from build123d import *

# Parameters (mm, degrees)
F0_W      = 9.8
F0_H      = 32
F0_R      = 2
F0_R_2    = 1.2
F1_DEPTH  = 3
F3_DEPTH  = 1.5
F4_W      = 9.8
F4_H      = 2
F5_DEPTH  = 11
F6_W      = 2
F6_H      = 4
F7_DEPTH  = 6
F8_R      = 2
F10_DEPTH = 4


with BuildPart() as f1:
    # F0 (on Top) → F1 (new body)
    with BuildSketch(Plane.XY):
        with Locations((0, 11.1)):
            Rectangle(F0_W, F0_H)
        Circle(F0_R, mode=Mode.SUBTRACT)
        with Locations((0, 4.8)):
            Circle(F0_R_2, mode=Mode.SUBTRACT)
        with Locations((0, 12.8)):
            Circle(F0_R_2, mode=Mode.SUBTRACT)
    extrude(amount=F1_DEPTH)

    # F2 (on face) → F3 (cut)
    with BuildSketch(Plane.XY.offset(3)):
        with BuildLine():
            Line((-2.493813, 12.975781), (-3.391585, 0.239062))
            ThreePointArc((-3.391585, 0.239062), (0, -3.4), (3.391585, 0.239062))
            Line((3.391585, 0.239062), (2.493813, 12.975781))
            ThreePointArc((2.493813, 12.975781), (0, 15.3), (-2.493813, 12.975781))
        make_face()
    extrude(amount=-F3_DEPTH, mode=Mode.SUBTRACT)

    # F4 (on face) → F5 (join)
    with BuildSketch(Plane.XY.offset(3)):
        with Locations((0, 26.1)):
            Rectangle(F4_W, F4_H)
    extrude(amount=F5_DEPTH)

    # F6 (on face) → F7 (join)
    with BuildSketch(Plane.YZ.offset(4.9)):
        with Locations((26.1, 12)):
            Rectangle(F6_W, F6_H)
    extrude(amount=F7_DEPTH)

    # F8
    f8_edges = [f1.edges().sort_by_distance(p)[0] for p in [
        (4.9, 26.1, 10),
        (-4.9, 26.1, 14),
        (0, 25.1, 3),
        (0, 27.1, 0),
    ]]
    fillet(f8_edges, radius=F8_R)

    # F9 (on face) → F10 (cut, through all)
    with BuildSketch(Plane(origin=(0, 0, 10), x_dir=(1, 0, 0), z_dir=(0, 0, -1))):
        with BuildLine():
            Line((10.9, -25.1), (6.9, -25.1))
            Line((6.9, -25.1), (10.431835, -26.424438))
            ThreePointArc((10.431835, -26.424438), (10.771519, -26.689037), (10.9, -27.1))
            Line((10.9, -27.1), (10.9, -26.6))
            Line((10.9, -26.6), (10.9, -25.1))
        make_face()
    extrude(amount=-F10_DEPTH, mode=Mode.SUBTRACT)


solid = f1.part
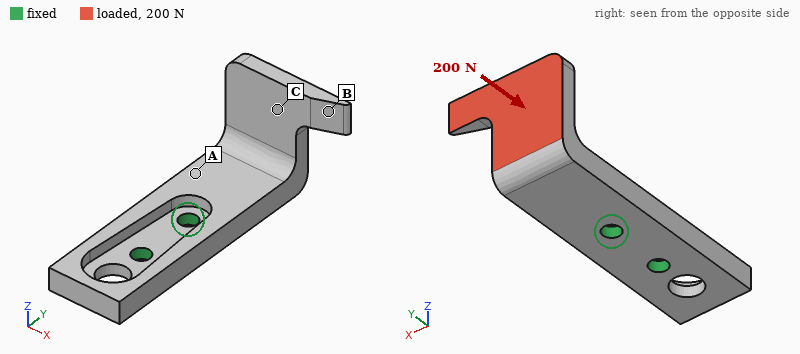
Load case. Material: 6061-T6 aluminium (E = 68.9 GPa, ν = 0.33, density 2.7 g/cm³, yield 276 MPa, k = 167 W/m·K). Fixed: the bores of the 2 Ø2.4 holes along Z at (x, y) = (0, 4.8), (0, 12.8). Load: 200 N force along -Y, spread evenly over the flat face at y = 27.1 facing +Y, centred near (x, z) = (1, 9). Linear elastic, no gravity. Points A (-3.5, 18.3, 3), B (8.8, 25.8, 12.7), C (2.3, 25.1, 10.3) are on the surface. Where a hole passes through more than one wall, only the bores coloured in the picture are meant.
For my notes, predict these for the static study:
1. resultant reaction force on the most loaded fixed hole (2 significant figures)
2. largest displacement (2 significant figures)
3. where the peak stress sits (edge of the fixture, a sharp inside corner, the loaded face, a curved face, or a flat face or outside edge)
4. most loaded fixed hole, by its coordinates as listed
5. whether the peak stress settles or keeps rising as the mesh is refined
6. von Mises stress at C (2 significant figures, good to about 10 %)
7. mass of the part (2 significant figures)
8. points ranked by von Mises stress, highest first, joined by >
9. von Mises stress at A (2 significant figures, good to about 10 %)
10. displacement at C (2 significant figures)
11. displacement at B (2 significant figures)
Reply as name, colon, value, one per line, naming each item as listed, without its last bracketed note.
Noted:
resultant reaction force on the most loaded fixed hole: 220 N
largest displacement: 0.35 mm
where the peak stress sits: edge of the fixture
most loaded fixed hole, by its coordinates as listed: (0, 4.8)
whether the peak stress settles or keeps rising as the mesh is refined: keeps rising
von Mises stress at C: 41 MPa
mass of the part: 2.7 g
points ranked by von Mises stress, highest first, joined by >: A > C > B
von Mises stress at A: 110 MPa
displacement at C: 0.21 mm
displacement at B: 0.30 mm
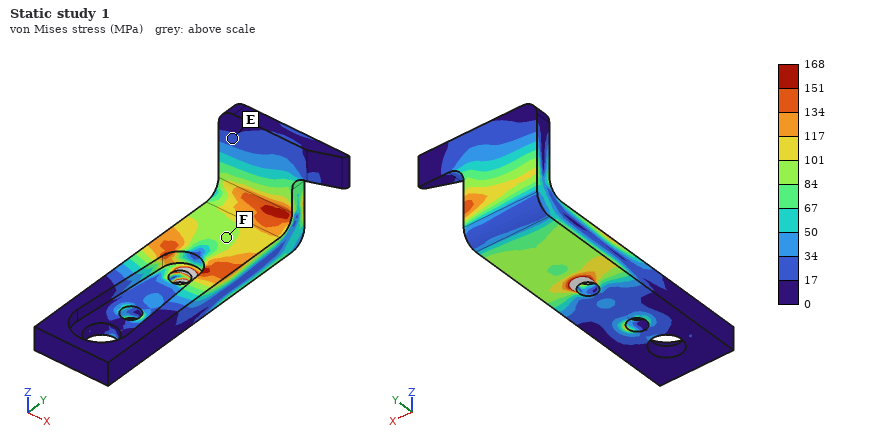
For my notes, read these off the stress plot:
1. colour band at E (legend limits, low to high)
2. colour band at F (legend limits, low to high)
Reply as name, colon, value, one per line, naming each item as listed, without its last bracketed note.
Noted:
colour band at E: 17 to 34 MPa
colour band at F: 84 to 101 MPa
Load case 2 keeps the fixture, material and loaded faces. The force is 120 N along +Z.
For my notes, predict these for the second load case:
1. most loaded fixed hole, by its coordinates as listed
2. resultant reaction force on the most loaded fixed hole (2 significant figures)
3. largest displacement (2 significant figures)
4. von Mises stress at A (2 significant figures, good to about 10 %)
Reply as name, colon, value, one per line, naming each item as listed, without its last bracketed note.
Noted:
most loaded fixed hole, by its coordinates as listed: (0, 12.8)
resultant reaction force on the most loaded fixed hole: 280 N
largest displacement: 0.22 mm
von Mises stress at A: 83 MPa
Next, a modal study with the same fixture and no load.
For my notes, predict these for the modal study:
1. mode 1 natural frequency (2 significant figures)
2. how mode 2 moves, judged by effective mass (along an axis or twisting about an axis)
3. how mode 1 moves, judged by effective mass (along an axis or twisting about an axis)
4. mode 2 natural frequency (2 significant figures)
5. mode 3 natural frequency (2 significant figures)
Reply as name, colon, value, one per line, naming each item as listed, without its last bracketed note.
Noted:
mode 1 natural frequency: 4300 Hz
how mode 2 moves, judged by effective mass: along X
how mode 1 moves, judged by effective mass: along Z
mode 2 natural frequency: 6200 Hz
mode 3 natural frequency: 11 kHz
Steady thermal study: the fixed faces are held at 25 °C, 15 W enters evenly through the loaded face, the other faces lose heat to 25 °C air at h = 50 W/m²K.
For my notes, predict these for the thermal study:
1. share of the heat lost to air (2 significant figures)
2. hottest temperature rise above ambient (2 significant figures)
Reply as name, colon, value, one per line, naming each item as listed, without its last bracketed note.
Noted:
share of the heat lost to air: 7.4 %
hottest temperature rise above ambient: 76 K
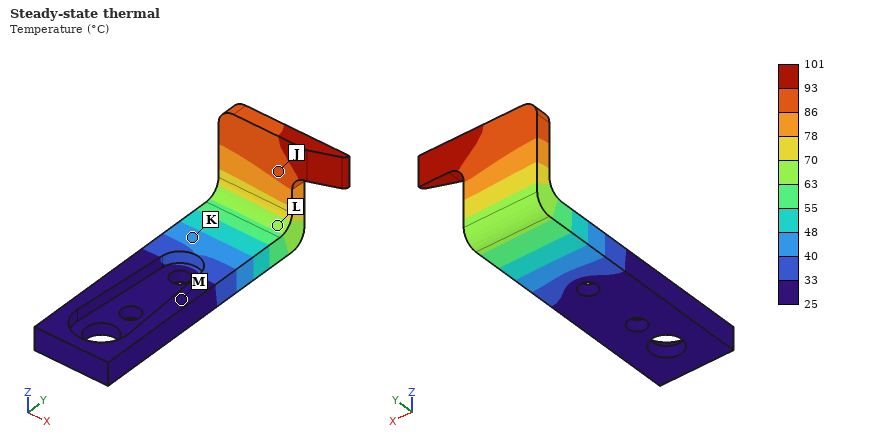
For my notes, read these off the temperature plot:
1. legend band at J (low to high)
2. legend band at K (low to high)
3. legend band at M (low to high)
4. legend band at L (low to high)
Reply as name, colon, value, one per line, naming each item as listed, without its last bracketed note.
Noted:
legend band at J: 86 to 93 °C
legend band at K: 40 to 48 °C
legend band at M: 25 to 33 °C
legend band at L: 63 to 70 °C
